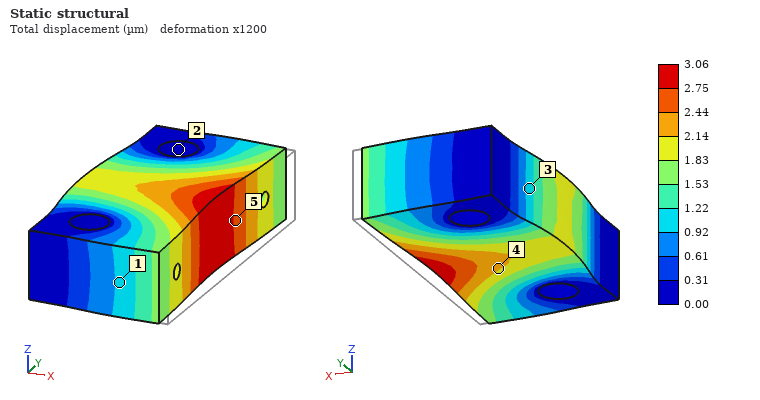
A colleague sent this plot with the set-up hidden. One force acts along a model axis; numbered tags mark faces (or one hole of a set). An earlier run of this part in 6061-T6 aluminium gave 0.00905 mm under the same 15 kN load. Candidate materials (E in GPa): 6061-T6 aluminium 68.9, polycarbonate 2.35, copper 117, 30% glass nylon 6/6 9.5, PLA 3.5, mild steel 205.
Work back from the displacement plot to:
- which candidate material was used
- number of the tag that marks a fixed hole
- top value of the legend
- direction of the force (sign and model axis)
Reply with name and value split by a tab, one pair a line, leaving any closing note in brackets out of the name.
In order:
which candidate material was used	mild steel
number of the tag that marks a fixed hole	2
top value of the legend	3.06 µm
direction of the force	-X
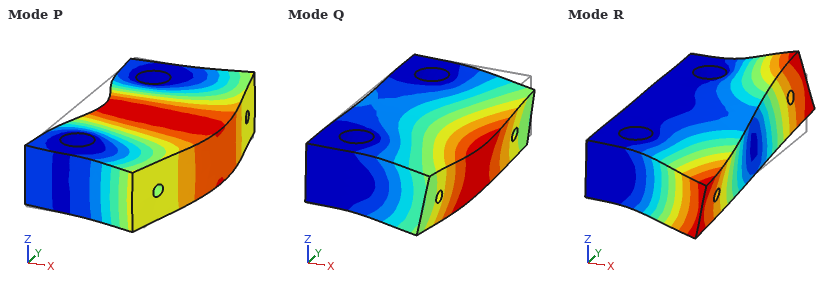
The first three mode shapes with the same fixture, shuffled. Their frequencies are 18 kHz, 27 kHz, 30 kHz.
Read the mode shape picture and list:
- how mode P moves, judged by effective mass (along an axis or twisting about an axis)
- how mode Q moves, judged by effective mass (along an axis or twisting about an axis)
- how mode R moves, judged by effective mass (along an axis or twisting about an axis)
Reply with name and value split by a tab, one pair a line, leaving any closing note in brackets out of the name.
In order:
how mode P moves, judged by effective mass	along X
how mode Q moves, judged by effective mass	along Z
how mode R moves, judged by effective mass	twisting about X
